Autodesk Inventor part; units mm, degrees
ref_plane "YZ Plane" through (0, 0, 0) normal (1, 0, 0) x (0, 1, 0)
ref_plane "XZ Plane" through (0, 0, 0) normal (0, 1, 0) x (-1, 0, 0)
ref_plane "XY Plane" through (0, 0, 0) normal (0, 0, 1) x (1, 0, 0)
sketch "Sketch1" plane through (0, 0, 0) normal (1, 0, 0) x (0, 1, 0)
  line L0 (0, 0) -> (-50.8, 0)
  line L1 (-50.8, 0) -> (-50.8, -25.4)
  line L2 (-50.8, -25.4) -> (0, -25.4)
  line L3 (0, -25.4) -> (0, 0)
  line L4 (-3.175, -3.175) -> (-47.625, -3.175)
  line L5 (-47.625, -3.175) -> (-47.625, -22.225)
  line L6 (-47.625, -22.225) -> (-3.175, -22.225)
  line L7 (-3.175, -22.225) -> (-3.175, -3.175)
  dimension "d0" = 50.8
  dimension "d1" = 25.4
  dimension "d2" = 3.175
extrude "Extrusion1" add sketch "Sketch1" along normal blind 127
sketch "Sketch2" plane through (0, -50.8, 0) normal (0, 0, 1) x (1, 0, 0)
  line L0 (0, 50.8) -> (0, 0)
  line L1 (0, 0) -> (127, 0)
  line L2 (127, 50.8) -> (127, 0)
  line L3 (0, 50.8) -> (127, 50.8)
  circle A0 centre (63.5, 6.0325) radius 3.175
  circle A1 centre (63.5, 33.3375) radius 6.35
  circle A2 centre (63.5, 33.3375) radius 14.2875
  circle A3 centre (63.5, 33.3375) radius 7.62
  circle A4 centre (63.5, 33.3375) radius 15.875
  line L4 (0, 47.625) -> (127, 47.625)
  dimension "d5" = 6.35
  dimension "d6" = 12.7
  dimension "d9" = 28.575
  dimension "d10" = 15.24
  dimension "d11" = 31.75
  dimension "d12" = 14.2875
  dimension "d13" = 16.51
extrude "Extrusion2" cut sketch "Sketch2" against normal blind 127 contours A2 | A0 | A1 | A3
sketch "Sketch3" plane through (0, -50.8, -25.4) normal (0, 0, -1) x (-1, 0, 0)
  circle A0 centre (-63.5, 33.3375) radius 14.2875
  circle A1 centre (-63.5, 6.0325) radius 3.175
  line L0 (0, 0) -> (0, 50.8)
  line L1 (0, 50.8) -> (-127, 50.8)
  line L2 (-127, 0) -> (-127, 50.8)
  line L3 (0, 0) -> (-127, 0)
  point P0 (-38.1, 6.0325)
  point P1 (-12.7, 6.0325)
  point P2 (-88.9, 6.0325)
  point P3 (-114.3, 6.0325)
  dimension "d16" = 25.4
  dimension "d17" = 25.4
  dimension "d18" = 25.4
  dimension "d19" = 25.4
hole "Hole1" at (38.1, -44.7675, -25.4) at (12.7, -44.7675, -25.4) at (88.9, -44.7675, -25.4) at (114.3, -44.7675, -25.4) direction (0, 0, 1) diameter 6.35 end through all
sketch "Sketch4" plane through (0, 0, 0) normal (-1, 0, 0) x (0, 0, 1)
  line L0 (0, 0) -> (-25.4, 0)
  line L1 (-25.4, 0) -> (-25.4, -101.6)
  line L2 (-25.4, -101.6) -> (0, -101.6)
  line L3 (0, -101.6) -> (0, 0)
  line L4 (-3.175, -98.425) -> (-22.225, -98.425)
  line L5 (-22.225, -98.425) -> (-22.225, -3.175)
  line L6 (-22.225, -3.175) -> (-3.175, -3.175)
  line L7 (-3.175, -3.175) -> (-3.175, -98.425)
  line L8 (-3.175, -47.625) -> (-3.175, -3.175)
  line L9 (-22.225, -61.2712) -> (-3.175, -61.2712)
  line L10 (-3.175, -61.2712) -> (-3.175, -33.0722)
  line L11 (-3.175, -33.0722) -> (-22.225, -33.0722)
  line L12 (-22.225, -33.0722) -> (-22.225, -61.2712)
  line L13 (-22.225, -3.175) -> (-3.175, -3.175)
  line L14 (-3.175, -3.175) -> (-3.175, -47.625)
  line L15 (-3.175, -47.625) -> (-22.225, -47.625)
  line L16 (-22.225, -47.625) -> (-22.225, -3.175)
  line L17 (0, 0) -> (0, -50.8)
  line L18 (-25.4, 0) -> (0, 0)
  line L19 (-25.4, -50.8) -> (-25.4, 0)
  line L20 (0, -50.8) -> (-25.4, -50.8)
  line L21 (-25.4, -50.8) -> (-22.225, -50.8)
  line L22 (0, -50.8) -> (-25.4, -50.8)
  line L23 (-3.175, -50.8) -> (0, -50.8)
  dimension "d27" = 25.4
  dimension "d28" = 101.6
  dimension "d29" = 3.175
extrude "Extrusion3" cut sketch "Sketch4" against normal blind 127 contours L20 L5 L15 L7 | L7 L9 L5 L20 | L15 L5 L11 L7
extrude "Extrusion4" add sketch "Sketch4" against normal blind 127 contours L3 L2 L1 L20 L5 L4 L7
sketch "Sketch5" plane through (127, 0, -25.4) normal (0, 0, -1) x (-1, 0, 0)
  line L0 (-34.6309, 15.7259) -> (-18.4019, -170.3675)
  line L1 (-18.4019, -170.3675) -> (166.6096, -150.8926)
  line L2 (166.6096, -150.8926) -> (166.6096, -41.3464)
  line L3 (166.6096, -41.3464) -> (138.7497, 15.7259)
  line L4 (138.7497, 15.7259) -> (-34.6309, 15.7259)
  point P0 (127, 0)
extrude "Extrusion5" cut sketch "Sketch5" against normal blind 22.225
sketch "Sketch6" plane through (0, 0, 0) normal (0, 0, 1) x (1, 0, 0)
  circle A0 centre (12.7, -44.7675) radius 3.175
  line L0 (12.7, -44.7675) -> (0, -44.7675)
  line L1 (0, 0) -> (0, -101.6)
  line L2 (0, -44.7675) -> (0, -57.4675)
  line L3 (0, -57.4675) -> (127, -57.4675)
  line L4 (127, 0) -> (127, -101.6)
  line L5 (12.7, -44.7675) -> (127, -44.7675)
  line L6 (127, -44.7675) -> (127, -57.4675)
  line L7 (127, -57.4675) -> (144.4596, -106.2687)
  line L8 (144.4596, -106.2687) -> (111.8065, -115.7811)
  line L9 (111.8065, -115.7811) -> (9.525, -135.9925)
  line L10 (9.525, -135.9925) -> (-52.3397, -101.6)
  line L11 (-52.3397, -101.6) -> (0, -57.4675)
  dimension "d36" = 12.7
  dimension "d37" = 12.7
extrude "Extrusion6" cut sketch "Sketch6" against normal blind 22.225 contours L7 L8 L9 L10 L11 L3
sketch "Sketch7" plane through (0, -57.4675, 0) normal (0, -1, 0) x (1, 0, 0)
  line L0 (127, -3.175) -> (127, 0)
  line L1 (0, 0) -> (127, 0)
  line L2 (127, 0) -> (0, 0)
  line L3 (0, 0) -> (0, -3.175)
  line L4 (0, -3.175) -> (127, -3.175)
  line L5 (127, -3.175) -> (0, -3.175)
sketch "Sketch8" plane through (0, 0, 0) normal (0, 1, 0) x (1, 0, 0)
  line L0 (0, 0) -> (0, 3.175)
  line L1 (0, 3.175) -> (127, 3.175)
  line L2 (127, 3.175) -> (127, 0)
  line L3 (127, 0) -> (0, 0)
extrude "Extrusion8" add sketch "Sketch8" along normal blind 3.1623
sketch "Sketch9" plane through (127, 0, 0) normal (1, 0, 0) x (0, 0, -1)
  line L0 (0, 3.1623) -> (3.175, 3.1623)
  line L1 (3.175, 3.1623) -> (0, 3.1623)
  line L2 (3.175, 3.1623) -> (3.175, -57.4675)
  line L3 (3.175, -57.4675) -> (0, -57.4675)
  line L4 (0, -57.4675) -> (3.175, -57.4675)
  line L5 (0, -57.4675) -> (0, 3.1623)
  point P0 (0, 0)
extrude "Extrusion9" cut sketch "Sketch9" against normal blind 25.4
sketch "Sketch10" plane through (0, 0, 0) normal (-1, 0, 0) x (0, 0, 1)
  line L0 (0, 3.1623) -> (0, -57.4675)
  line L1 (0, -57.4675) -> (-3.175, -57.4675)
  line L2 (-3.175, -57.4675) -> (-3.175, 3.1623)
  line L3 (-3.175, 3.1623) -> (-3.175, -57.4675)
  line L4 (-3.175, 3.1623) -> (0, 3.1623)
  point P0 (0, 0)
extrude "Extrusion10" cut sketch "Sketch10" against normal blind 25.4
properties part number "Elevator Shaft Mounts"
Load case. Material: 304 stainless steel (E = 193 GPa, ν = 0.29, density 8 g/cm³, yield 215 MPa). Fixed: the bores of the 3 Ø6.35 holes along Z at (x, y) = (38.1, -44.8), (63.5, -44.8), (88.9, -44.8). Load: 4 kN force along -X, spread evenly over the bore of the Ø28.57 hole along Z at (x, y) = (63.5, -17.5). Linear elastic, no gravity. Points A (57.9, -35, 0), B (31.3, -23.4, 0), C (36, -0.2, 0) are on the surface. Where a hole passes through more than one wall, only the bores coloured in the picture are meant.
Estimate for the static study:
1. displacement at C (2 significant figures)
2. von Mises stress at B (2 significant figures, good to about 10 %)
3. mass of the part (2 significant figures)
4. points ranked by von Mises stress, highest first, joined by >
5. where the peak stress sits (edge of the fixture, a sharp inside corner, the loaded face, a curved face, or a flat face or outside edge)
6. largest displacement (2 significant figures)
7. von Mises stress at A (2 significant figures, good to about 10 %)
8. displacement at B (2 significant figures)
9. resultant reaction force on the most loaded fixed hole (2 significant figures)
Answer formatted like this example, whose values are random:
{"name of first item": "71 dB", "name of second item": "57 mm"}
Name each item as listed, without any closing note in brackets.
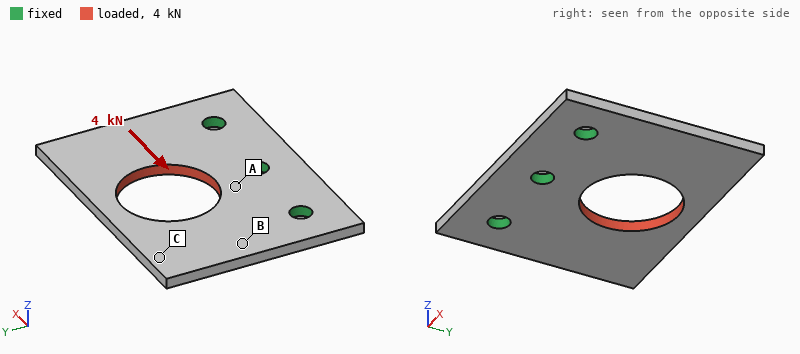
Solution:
{"displacement at C": "24 µm", "von Mises stress at B": "25 MPa", "mass of the part": "99 g", "points ranked by von Mises stress, highest first, joined by >": "A > B > C", "where the peak stress sits": "edge of the fixture", "largest displacement": "28 µm", "von Mises stress at A": "61 MPa", "displacement at B": "11 µm", "resultant reaction force on the most loaded fixed hole": "2.1 kN"}
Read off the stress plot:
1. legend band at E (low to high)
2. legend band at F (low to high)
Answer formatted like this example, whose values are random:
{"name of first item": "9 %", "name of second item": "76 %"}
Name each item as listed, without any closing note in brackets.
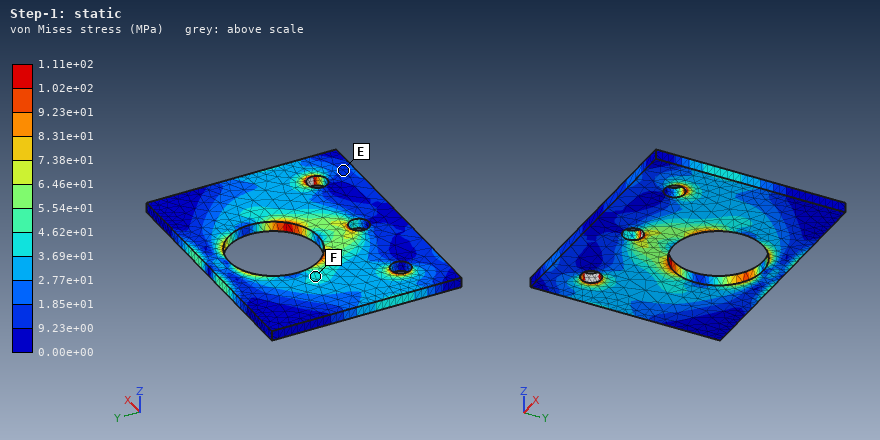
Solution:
{"legend band at E": "9.23e+00 to 1.85e+01 MPa", "legend band at F": "3.69e+01 to 4.62e+01 MPa"}
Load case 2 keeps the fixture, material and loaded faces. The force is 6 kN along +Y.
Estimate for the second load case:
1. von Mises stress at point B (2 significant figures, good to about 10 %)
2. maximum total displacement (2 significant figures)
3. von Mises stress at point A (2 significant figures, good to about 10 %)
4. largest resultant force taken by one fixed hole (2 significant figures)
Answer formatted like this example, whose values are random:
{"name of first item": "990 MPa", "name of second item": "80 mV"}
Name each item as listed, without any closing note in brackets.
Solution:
{"von Mises stress at point B": "12 MPa", "maximum total displacement": "18 µm", "von Mises stress at point A": "25 MPa", "largest resultant force taken by one fixed hole": "2.3 kN"}
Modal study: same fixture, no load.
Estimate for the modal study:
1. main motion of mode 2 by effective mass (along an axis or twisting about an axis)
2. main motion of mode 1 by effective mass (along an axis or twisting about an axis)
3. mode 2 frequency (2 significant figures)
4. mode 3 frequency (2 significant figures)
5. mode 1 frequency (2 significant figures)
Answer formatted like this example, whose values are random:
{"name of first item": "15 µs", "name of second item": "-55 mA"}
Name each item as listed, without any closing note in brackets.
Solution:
{"main motion of mode 2 by effective mass": "twisting about Y", "main motion of mode 1 by effective mass": "along Z", "mode 2 frequency": "1800 Hz", "mode 3 frequency": "4000 Hz", "mode 1 frequency": "1100 Hz"}
